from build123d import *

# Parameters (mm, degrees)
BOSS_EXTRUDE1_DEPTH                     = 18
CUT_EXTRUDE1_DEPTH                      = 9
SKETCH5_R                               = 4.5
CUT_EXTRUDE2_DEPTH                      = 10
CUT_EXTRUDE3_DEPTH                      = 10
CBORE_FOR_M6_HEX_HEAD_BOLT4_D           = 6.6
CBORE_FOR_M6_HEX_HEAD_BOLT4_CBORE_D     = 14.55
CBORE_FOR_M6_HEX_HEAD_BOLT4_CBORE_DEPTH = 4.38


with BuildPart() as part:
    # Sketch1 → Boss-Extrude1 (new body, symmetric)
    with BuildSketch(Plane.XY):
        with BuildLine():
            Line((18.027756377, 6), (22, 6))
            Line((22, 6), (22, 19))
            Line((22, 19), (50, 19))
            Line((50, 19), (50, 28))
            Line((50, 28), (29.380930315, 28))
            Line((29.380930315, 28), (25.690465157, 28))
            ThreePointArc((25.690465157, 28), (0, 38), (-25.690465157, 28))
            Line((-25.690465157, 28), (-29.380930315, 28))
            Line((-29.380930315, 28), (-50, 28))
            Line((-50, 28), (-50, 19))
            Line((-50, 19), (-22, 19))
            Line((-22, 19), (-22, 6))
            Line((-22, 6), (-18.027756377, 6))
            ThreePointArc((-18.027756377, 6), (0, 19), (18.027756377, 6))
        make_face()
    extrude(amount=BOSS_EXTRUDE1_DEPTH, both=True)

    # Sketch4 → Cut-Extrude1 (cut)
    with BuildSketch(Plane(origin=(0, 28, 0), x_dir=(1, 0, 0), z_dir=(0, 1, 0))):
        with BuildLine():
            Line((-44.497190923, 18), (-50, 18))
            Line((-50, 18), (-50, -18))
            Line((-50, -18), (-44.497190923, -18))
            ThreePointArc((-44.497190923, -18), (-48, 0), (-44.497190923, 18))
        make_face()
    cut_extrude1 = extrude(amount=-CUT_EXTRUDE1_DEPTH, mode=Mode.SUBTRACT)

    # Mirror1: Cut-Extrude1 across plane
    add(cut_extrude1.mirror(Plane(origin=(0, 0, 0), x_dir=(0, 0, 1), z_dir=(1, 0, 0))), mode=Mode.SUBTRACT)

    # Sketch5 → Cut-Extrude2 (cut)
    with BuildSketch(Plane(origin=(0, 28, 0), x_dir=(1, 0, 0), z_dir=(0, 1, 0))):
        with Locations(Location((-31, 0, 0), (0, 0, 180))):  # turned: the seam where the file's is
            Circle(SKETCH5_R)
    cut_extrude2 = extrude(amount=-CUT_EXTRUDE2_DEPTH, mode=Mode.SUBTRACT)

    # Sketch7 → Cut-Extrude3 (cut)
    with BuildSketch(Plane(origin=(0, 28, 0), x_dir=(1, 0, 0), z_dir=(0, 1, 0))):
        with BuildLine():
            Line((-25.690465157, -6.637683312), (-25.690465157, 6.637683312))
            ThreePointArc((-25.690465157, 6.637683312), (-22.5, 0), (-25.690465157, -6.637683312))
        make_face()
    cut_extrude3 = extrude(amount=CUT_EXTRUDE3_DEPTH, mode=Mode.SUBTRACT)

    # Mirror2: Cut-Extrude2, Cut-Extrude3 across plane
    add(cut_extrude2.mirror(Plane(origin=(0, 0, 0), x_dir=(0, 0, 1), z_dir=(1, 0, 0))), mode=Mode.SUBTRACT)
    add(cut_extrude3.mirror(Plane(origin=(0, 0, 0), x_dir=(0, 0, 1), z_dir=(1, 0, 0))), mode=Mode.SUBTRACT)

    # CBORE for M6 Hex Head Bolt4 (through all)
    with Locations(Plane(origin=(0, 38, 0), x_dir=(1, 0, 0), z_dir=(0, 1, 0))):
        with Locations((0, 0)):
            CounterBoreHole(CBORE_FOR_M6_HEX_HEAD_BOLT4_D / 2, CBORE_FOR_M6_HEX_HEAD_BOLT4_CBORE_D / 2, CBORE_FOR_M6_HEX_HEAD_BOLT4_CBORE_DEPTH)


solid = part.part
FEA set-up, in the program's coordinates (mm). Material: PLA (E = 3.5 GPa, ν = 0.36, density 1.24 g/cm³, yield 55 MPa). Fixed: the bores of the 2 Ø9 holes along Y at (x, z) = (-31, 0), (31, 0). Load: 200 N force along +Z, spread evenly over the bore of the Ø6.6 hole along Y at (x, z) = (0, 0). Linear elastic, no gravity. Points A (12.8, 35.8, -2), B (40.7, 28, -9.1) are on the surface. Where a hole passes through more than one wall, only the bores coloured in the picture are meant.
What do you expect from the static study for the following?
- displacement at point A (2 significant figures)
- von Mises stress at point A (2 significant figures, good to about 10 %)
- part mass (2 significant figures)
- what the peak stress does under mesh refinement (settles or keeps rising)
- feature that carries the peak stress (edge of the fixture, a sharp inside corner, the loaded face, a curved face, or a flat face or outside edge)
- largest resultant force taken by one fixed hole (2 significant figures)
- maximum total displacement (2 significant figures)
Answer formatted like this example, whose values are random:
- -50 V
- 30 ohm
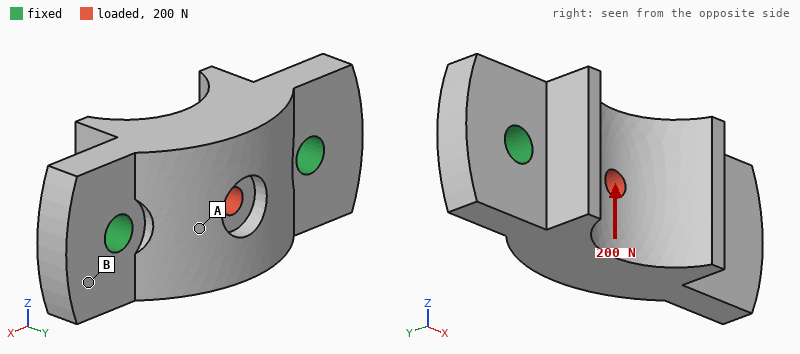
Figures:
- 8.8 µm
- 0.42 MPa
- 61 g
- keeps rising
- edge of the fixture
- 100 N
- 12 µm
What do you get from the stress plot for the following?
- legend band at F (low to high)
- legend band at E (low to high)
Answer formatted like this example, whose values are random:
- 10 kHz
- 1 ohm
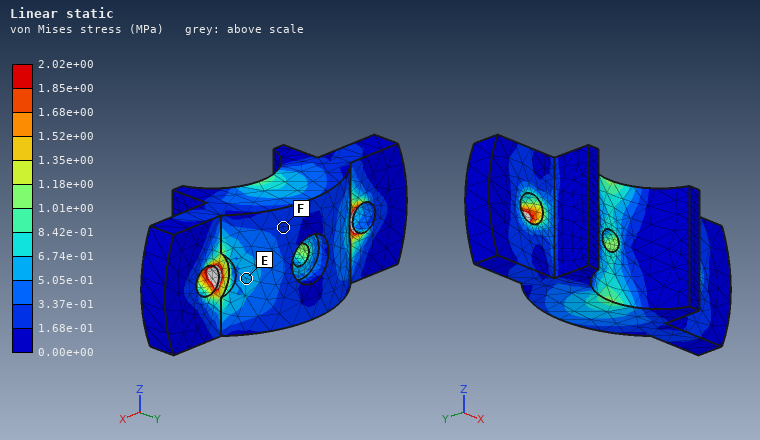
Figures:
- 1.68e-01 to 3.37e-01 MPa
- 5.05e-01 to 6.74e-01 MPa
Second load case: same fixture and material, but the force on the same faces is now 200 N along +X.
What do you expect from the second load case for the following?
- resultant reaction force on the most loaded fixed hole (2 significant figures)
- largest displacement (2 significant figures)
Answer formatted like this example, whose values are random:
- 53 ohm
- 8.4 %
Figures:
- 100 N
- 3.4 µm
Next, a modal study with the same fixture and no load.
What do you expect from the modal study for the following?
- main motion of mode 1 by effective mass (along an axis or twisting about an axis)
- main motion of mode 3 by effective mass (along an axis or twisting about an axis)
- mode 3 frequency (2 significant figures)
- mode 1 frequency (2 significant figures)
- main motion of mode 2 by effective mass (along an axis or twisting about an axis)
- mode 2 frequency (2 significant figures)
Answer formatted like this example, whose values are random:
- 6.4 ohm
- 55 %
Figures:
- twisting about X
- along Z
- 4900 Hz
- 3000 Hz
- along Y
- 3700 Hz
